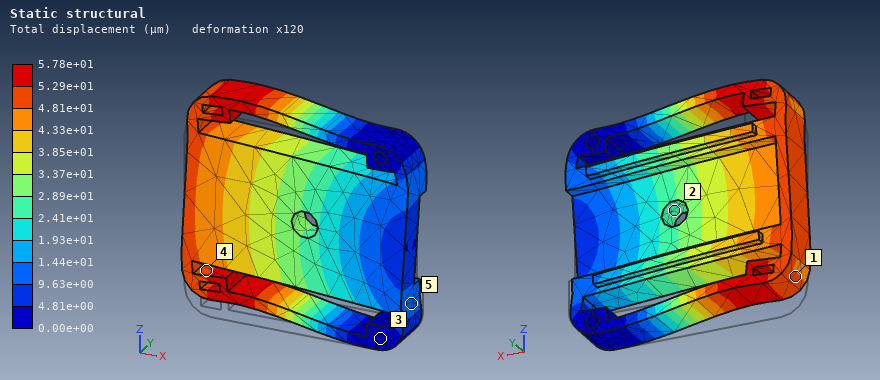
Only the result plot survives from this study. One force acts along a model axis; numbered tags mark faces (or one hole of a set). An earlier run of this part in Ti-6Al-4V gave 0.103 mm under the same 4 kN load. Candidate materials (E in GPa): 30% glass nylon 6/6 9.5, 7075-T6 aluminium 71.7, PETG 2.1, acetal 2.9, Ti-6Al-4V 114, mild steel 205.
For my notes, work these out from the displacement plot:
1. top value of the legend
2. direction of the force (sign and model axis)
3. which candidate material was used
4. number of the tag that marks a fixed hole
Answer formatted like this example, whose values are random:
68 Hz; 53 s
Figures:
5.78e+01 µm; +Z; mild steel; 3
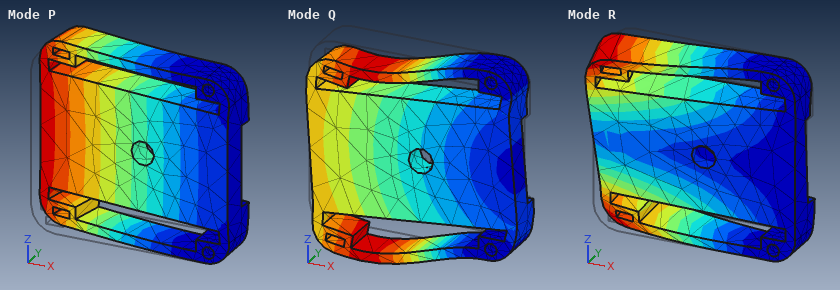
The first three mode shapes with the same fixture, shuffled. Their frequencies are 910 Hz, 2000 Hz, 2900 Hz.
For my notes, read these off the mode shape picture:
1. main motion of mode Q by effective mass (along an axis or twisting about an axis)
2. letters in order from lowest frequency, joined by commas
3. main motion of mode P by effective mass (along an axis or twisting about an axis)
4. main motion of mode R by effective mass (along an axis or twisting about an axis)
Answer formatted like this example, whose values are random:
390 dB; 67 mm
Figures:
along Z; P, Q, R; along Y; twisting about X
